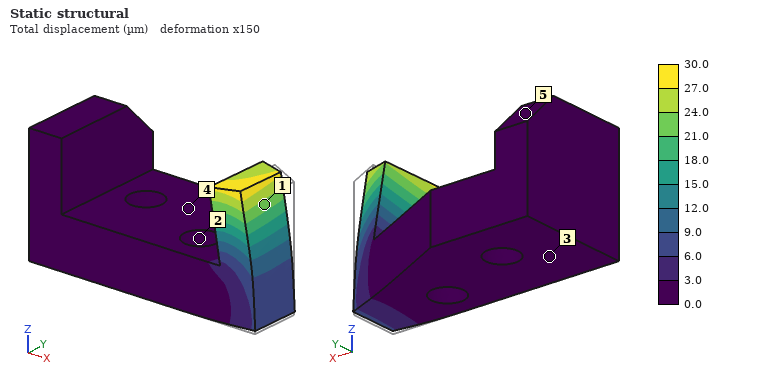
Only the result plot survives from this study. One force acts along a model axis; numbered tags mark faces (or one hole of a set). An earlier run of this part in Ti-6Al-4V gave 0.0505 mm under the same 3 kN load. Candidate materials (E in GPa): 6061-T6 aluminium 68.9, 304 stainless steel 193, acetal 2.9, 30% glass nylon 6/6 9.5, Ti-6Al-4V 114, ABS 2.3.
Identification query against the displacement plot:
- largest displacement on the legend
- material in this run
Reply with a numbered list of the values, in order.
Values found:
1. 30.0 µm
2. 304 stainless steel
